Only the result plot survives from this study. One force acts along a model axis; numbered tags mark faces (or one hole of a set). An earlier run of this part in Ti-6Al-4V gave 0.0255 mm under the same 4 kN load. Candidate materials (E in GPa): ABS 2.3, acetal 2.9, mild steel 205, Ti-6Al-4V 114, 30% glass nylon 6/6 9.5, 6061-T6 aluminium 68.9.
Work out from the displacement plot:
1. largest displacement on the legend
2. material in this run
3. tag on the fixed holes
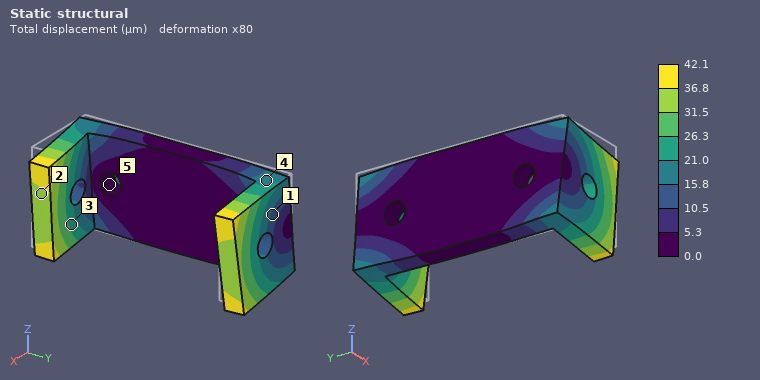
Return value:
42.1 µm
6061-T6 aluminium
5
